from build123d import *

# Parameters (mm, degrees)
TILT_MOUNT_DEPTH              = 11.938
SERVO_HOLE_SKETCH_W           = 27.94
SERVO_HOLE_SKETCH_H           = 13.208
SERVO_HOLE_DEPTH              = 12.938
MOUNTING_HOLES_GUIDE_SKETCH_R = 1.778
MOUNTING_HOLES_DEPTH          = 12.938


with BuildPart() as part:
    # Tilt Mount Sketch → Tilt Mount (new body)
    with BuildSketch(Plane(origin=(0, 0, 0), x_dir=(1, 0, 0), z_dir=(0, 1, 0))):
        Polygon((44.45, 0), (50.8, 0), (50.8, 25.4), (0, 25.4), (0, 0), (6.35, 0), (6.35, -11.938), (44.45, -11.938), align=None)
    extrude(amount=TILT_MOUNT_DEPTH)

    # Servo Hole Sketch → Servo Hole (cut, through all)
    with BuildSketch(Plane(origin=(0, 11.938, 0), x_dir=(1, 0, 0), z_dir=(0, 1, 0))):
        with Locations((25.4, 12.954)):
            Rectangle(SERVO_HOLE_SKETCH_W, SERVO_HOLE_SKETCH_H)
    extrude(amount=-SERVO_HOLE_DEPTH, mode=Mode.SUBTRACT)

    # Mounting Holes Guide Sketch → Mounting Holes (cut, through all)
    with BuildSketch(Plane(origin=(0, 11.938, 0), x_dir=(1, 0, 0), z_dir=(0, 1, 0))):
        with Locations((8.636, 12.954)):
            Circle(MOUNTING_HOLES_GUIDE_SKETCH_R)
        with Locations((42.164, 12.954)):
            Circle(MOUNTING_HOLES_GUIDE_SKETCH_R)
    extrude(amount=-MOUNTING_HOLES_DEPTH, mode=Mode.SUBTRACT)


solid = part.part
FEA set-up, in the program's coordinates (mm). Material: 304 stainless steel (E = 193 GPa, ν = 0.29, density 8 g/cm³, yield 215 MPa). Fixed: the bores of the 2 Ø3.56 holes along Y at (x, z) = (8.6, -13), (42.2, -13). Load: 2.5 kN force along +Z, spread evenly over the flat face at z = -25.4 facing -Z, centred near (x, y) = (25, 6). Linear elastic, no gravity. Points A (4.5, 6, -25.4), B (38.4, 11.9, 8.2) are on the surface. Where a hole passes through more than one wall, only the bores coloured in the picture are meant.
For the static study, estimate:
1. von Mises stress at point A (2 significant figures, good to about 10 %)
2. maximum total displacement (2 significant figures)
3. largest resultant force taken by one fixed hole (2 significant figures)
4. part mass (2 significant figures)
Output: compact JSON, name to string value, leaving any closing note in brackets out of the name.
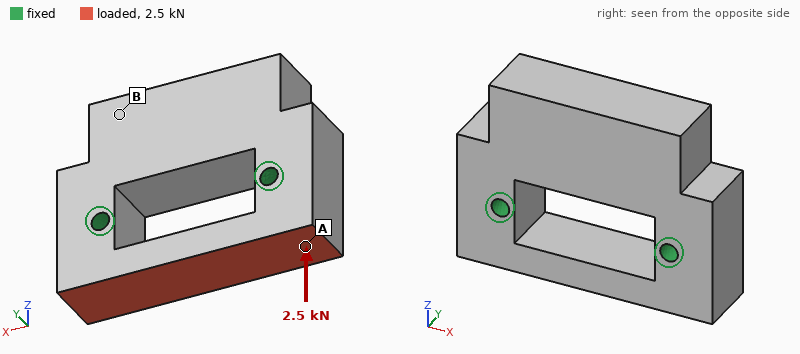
{"von Mises stress at point A": "11 MPa", "maximum total displacement": "6.2 µm", "largest resultant force taken by one fixed hole": "1.3 kN", "part mass": "130 g"}
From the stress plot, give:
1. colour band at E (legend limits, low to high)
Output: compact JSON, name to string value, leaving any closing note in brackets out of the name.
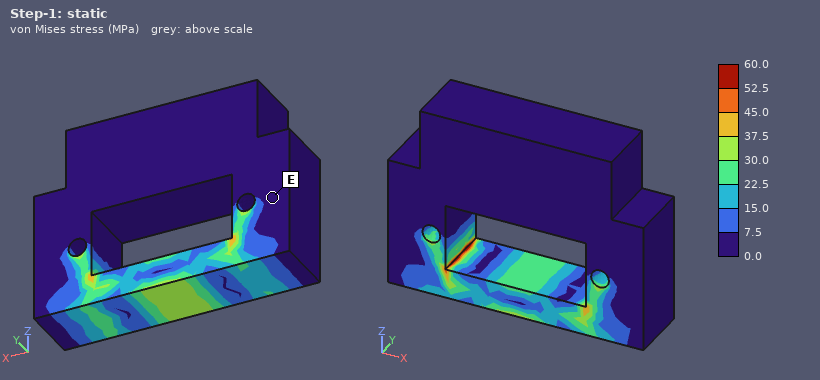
{"colour band at E": "0.0 to 7.5 MPa"}
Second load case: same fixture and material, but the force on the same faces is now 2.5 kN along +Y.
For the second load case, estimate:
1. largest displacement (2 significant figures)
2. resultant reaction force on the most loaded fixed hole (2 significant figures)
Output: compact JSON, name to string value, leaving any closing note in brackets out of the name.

{"largest displacement": "9.9 µm", "resultant reaction force on the most loaded fixed hole": "1.3 kN"}
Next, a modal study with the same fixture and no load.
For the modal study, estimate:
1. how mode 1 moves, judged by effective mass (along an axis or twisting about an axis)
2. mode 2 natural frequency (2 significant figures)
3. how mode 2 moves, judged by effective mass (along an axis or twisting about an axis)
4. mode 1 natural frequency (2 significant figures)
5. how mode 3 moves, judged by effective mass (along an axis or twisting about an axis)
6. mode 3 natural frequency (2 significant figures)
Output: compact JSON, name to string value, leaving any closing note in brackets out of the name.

{"how mode 1 moves, judged by effective mass": "along Y", "mode 2 natural frequency": "14 kHz", "how mode 2 moves, judged by effective mass": "along X", "mode 1 natural frequency": "8900 Hz", "how mode 3 moves, judged by effective mass": "twisting about Z", "mode 3 natural frequency": "19 kHz"}
